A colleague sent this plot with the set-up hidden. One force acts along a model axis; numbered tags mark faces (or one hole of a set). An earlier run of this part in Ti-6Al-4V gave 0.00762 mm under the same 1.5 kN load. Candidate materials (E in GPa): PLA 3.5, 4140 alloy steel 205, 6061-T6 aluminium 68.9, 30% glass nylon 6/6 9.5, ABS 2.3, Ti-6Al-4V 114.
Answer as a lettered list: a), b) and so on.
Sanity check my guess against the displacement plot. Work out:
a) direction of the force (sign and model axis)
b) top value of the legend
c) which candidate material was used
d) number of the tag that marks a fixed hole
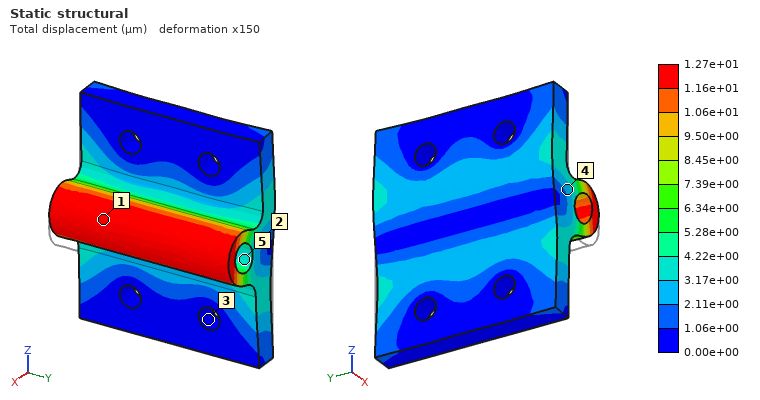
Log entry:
a) +Z
b) 1.27e+01 µm
c) 6061-T6 aluminium
d) 3
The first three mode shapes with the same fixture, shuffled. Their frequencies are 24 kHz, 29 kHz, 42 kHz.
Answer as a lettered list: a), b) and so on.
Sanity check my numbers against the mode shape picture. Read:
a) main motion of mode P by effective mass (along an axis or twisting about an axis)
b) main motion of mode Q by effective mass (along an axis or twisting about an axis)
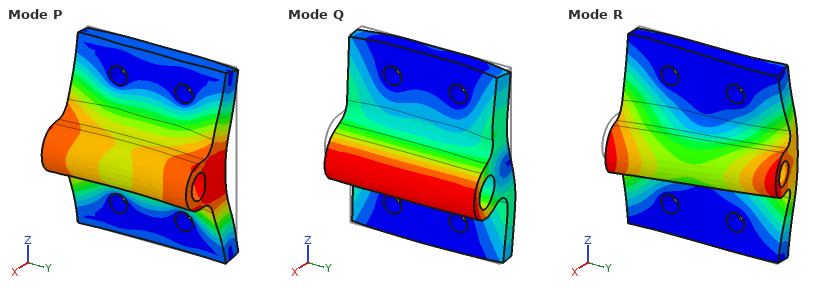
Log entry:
a) along X
b) along Z
